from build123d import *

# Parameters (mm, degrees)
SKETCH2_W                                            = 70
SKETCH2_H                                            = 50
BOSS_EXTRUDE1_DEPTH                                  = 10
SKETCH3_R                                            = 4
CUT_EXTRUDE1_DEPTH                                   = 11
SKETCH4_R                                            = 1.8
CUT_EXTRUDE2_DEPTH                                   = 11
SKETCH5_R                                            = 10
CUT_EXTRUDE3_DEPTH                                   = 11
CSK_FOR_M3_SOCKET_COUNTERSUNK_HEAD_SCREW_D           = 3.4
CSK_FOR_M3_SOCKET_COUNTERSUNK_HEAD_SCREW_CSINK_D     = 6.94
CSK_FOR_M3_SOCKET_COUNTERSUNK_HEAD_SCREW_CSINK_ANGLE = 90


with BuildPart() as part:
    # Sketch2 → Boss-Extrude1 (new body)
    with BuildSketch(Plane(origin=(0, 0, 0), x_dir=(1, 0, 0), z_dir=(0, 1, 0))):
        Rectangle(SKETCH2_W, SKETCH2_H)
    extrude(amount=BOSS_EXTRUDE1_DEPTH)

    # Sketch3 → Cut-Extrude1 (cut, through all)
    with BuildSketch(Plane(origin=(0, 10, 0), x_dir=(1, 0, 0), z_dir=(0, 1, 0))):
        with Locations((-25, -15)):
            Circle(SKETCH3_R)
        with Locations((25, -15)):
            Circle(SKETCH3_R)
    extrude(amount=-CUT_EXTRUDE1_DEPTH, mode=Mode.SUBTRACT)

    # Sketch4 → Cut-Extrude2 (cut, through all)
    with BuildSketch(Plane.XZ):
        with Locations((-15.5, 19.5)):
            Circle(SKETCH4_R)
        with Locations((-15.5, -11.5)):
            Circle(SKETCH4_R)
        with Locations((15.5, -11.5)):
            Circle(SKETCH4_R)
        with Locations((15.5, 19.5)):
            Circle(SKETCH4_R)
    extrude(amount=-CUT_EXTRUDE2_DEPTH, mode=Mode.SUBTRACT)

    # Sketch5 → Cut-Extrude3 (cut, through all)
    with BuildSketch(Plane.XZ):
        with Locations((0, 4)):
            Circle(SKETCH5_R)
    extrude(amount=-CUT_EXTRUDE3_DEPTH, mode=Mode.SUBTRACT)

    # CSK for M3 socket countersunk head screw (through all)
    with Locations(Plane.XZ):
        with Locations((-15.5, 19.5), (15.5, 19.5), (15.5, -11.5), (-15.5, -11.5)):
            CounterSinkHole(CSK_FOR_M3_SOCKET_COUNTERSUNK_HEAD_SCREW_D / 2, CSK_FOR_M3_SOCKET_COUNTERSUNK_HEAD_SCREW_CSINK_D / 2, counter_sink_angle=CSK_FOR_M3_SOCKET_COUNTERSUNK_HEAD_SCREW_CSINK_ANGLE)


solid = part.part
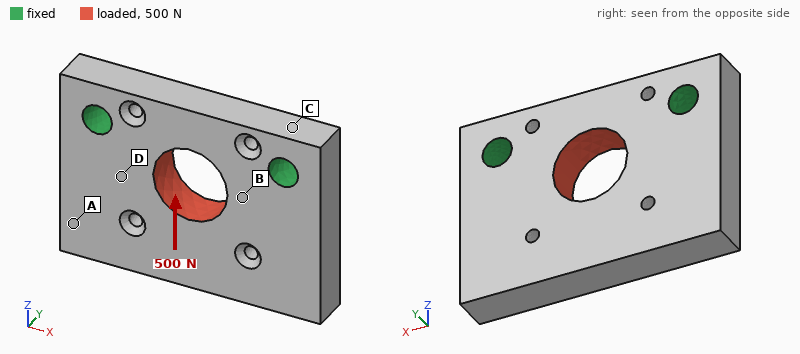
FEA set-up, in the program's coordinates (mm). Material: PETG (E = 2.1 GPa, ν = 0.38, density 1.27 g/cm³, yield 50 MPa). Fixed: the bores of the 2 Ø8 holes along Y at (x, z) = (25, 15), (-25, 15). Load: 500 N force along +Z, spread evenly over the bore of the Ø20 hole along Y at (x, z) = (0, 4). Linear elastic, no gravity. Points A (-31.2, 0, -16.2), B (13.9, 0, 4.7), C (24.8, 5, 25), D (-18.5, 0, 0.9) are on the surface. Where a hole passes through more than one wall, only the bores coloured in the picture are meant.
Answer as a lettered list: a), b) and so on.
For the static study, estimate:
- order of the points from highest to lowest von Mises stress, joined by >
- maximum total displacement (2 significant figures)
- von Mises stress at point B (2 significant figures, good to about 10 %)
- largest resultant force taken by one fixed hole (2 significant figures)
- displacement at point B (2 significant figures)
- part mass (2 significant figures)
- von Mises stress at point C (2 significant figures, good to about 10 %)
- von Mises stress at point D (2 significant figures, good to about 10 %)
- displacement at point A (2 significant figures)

a) B > D > C > A
b) 29 µm
c) 1.6 MPa
d) 260 N
e) 14 µm
f) 39 g
g) 0.86 MPa
h) 1.3 MPa
i) 6.9 µm
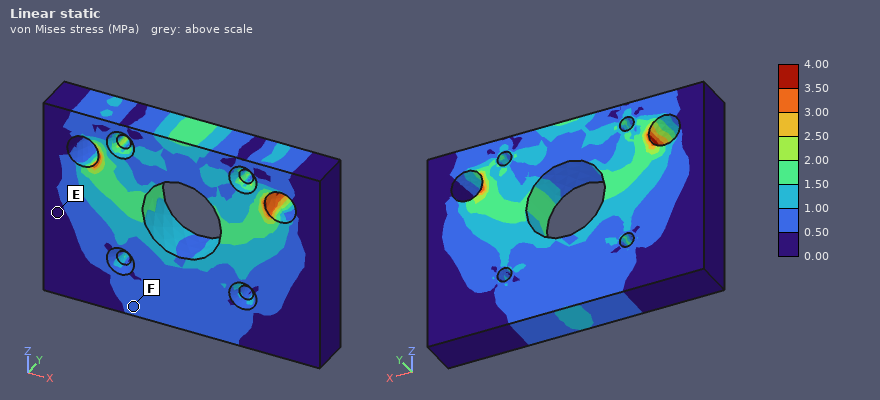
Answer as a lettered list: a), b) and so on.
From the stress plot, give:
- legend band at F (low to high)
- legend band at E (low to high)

a) 0.50 to 1.00 MPa
b) 0.00 to 0.50 MPa
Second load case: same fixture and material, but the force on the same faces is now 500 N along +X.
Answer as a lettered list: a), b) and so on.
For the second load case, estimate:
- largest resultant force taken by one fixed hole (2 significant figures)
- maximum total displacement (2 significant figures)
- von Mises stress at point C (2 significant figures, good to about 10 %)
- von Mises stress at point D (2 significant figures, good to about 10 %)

a) 260 N
b) 29 µm
c) 0.50 MPa
d) 1.2 MPa
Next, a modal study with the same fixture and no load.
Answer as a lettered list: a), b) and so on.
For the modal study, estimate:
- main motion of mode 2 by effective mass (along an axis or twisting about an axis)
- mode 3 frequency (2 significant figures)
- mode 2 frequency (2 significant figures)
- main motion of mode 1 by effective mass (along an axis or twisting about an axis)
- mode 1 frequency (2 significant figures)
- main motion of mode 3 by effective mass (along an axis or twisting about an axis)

a) twisting about Z
b) 3200 Hz
c) 1900 Hz
d) along Y
e) 1100 Hz
f) along X
